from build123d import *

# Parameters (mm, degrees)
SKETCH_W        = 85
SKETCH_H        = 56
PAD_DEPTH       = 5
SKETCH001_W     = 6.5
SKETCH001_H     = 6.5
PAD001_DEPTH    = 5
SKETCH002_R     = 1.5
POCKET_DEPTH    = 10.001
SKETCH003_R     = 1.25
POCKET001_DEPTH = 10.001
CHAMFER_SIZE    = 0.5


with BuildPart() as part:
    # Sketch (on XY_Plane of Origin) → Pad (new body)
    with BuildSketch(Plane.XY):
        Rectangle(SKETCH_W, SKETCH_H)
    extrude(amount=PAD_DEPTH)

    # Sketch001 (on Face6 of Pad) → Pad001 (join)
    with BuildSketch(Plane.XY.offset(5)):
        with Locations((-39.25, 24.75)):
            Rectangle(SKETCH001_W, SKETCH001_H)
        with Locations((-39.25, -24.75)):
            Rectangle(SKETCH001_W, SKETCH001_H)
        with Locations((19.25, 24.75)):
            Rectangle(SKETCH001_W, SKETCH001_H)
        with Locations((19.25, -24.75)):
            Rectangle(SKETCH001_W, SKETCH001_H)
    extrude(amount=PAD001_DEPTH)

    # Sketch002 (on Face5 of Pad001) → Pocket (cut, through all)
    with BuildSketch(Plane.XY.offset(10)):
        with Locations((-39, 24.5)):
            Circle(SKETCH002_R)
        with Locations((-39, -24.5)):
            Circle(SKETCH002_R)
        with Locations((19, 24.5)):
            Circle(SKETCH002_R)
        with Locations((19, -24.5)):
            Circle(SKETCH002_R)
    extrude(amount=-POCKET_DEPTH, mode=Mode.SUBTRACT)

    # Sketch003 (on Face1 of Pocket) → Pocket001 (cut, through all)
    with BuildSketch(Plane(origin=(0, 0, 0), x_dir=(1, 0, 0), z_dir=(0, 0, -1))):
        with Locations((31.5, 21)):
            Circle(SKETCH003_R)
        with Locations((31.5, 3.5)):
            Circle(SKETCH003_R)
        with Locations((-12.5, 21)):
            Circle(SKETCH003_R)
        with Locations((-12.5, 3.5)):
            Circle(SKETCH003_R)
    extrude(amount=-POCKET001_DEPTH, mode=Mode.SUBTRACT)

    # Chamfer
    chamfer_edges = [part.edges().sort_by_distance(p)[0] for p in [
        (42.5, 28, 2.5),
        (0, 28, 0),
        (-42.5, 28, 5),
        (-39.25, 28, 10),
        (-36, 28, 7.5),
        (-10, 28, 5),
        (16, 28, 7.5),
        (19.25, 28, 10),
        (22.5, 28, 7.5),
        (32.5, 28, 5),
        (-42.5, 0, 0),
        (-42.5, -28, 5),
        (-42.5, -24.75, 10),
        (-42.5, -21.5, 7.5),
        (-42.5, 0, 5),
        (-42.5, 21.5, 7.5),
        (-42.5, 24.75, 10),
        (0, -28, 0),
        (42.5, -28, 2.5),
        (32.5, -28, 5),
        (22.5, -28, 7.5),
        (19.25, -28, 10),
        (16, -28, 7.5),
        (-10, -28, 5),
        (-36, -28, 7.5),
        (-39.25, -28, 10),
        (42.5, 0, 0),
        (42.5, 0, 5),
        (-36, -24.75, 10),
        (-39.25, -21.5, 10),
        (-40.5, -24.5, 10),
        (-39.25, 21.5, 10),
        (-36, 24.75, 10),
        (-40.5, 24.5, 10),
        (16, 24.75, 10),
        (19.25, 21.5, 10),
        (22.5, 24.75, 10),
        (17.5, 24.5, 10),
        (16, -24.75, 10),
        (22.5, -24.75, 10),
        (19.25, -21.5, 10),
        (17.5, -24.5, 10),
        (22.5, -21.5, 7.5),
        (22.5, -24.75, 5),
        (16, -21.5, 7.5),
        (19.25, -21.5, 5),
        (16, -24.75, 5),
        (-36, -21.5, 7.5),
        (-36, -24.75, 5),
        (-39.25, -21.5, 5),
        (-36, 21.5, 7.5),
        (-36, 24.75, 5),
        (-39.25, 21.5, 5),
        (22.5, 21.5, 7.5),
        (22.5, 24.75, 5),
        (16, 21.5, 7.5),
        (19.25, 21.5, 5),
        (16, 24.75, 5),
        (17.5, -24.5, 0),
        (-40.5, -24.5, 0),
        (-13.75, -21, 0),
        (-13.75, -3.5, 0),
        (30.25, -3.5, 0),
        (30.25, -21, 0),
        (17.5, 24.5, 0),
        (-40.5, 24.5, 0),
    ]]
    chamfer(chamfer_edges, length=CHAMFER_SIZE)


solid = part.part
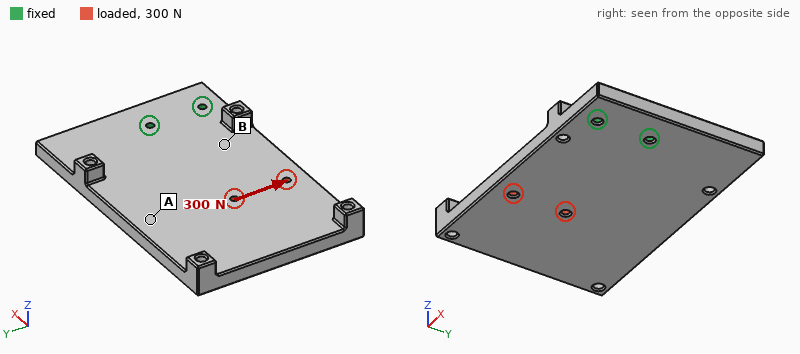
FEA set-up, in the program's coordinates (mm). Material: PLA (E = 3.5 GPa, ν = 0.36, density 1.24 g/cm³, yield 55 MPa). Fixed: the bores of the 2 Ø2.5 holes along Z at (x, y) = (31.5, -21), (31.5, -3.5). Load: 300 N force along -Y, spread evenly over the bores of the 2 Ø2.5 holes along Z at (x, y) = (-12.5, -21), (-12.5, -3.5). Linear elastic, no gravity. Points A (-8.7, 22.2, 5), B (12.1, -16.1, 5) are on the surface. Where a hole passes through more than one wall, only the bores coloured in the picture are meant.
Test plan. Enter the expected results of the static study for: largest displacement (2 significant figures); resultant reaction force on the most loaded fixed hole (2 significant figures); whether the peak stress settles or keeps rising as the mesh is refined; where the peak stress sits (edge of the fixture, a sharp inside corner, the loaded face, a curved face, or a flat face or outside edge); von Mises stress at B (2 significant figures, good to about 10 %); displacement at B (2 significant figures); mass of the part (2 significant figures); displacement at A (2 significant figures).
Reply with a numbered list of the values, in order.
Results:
1. 0.50 mm
2. 720 N
3. keeps rising
4. edge of the fixture
5. 5.4 MPa
6. 0.11 mm
7. 30 g
8. 0.31 mm
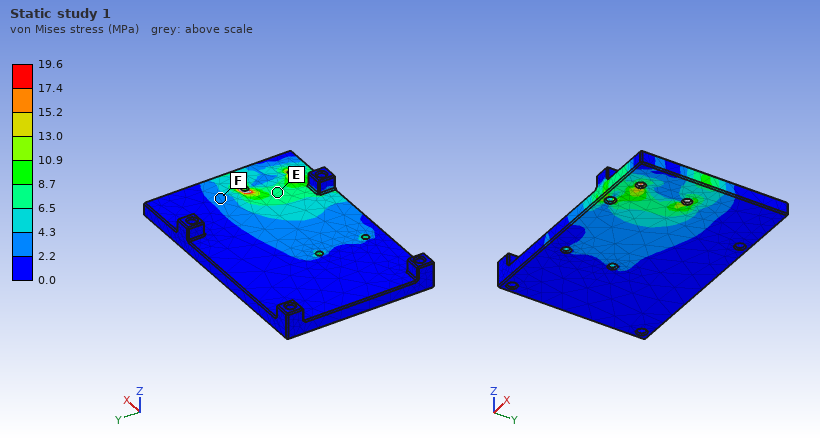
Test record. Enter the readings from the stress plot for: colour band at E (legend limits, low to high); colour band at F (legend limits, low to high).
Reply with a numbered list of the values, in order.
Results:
1. 6.5 to 8.7 MPa
2. 2.2 to 4.3 MPa
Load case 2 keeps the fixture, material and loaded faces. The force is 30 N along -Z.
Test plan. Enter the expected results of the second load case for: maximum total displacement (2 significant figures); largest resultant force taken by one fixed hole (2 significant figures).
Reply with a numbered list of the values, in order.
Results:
1. 1.2 mm
2. 15 N
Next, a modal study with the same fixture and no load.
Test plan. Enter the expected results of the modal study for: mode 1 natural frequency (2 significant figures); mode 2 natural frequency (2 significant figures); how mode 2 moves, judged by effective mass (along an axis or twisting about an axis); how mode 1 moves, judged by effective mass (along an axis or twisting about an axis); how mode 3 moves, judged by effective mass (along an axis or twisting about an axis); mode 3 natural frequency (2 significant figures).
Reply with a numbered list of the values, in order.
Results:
1. 210 Hz
2. 570 Hz
3. twisting about X
4. along Z
5. along Y
6. 970 Hz
